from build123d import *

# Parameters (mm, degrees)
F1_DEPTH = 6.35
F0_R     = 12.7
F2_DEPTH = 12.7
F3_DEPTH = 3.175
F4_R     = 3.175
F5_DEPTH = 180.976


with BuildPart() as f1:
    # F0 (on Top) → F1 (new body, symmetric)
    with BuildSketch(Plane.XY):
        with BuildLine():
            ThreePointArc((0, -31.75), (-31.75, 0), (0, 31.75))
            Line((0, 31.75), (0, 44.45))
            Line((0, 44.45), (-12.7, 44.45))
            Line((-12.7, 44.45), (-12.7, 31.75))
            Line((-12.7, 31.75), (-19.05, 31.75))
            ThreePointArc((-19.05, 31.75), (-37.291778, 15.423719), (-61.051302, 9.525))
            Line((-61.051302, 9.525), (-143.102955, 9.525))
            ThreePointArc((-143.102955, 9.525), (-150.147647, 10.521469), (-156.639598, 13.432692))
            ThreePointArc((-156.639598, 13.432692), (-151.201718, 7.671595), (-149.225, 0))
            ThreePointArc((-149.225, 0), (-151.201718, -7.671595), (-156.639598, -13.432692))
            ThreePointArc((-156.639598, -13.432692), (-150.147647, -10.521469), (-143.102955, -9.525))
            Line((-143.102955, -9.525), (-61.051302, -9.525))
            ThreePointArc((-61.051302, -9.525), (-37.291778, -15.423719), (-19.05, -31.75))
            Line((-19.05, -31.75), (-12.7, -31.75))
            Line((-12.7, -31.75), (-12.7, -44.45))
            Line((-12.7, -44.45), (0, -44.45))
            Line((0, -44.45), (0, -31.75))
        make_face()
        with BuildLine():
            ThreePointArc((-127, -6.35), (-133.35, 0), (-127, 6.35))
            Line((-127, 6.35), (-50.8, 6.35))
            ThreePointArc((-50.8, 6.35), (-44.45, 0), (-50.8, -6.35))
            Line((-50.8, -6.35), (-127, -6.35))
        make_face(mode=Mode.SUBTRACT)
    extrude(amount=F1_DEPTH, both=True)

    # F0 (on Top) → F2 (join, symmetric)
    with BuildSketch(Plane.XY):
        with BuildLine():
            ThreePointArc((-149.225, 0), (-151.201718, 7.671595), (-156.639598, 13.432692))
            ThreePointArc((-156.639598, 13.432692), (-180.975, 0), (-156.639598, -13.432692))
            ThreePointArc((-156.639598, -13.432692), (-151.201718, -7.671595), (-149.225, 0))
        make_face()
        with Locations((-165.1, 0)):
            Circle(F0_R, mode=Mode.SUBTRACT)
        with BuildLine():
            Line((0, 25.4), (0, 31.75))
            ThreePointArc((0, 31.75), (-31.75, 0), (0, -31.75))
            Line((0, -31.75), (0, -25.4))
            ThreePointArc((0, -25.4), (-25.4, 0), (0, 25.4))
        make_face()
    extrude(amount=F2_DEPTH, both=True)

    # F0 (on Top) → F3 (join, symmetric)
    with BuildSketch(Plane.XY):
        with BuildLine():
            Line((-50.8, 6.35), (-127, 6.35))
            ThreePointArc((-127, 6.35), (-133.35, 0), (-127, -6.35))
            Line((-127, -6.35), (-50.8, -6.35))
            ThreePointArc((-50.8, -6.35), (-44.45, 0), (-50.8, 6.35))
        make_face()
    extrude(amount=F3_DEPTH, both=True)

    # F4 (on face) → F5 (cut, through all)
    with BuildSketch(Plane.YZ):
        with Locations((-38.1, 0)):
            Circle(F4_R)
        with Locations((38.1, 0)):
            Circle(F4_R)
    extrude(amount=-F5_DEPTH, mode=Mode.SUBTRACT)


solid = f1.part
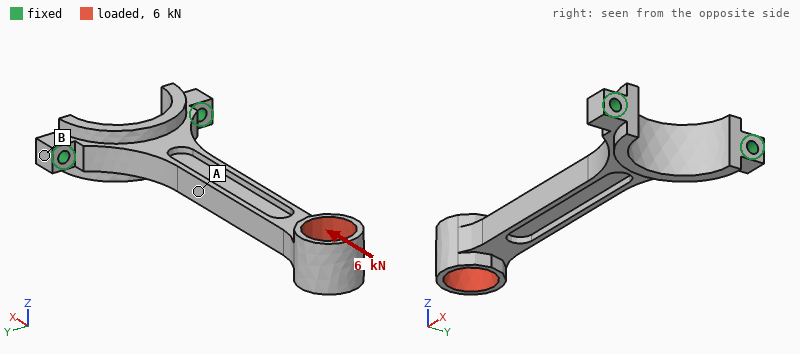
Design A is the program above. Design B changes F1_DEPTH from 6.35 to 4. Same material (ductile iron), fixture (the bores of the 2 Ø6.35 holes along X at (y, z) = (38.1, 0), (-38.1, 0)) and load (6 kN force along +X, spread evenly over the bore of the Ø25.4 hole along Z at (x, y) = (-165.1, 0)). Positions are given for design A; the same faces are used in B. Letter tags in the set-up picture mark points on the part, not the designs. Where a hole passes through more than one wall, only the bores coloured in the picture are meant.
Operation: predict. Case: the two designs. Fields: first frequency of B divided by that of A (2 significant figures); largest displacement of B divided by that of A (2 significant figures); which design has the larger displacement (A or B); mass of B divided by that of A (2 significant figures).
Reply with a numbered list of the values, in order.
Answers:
1. 0.67
2. 1.2
3. B
4. 0.83
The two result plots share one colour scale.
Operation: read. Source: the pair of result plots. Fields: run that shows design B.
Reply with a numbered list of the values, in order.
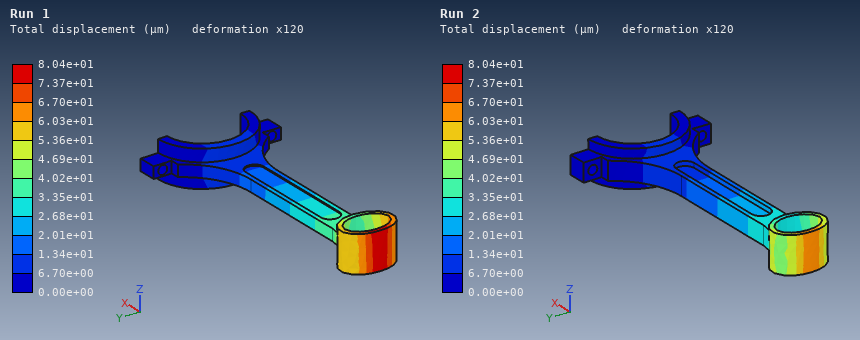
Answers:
1. Run 1
